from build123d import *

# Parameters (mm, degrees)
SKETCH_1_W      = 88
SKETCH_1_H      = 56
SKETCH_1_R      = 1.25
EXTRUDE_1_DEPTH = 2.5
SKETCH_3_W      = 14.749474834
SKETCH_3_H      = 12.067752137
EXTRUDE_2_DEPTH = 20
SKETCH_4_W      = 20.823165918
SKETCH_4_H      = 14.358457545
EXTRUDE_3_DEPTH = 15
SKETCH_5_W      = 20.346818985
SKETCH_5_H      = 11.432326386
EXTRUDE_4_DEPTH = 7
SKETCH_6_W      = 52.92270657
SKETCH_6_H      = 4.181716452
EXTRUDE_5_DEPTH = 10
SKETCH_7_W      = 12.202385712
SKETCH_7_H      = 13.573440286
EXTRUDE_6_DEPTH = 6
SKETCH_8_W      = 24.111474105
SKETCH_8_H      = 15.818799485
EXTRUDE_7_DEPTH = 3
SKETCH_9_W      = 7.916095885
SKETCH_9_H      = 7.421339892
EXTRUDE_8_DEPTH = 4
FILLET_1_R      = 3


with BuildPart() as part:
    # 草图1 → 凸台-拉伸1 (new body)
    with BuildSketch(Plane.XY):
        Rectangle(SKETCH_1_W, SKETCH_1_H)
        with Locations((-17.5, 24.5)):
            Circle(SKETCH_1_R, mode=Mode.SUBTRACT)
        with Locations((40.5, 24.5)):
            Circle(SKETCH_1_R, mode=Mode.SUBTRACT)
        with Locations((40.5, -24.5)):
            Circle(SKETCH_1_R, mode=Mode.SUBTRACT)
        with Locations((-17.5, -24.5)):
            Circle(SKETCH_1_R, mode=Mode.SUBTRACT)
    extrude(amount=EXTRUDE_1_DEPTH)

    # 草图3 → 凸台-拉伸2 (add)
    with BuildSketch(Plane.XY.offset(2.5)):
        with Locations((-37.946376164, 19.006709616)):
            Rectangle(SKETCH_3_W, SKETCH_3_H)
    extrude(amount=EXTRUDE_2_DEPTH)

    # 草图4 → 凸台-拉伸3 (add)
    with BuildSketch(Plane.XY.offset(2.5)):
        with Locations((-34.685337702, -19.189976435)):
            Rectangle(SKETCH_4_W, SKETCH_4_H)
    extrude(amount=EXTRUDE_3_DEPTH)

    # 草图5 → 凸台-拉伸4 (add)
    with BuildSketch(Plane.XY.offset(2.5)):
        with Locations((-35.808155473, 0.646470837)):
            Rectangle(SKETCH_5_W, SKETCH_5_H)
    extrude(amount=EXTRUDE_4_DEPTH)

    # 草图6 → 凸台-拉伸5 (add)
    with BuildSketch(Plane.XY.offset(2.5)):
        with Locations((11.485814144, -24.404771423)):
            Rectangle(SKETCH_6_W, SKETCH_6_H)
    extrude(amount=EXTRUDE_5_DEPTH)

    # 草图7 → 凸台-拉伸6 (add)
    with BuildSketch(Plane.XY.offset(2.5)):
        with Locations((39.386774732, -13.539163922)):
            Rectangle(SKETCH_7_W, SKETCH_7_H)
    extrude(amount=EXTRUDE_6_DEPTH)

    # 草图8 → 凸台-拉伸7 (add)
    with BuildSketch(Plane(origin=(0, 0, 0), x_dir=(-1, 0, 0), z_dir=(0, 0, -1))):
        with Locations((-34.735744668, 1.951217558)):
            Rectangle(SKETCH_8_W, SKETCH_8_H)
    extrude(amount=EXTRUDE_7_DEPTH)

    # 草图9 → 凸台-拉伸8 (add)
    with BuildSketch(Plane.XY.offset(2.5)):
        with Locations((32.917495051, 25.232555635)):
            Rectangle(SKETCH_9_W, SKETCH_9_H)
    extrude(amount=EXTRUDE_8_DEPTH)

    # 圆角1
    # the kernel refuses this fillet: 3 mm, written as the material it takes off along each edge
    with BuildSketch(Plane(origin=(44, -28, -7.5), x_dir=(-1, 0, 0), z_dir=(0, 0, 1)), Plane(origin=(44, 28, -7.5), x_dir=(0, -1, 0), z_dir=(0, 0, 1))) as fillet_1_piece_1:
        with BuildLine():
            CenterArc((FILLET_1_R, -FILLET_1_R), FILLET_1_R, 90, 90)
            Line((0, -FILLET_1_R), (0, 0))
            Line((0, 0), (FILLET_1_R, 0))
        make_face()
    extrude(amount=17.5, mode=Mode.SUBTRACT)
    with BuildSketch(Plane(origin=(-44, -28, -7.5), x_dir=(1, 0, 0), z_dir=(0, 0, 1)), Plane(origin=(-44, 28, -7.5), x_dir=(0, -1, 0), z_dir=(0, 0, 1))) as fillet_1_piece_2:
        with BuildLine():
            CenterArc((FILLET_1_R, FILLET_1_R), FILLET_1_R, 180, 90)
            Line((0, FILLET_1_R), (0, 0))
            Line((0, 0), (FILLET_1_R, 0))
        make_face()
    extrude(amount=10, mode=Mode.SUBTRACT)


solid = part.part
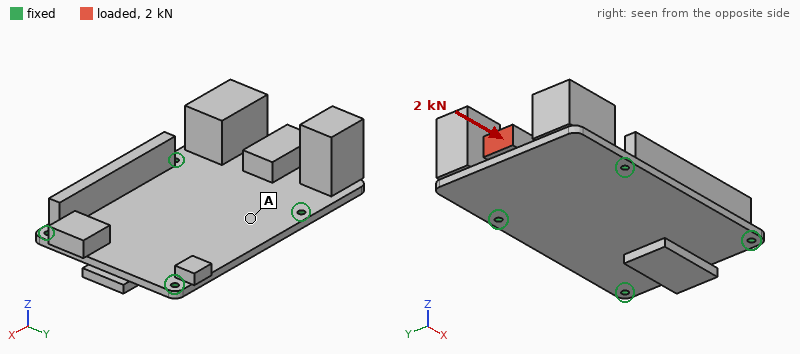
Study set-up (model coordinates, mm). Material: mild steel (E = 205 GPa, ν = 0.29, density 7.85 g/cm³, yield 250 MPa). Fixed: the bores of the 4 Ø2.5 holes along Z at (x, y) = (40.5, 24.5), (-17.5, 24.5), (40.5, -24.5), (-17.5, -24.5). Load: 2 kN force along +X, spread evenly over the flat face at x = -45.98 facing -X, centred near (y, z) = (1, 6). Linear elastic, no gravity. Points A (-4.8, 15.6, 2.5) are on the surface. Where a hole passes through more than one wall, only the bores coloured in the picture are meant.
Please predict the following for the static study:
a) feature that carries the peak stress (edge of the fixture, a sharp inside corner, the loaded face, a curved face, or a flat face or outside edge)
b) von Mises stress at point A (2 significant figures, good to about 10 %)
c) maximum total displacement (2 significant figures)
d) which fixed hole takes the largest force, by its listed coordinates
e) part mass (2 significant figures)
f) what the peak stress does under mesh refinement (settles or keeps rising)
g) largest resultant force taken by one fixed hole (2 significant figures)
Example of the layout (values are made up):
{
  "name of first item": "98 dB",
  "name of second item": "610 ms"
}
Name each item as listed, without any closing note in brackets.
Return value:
{
  "feature that carries the peak stress": "edge of the fixture",
  "von Mises stress at point A": "29 MPa",
  "maximum total displacement": "0.26 mm",
  "which fixed hole takes the largest force, by its listed coordinates": "(-17.5, 24.5)",
  "part mass": "210 g",
  "what the peak stress does under mesh refinement": "keeps rising",
  "largest resultant force taken by one fixed hole": "800 N"
}
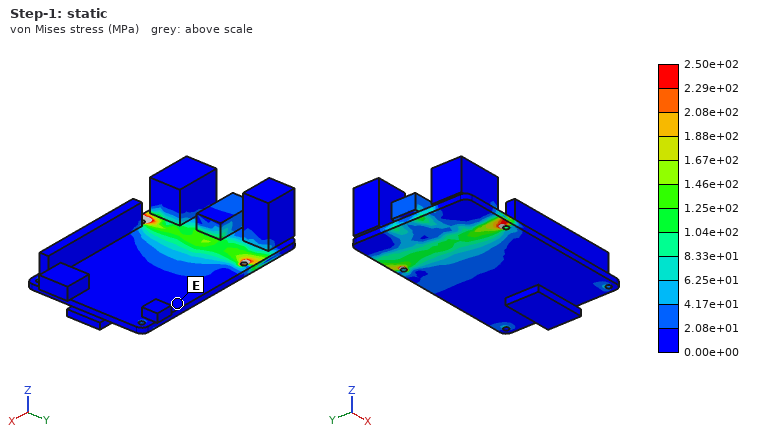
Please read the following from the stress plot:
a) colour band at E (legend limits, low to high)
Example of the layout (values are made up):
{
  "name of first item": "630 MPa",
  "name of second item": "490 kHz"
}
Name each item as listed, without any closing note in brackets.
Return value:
{
  "colour band at E": "0.00e+00 to 2.08e+01 MPa"
}
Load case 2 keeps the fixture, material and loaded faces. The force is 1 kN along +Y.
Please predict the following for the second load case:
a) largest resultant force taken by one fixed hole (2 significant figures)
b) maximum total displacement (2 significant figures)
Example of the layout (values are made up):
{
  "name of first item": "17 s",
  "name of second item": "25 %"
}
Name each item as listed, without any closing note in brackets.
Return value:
{
  "largest resultant force taken by one fixed hole": "750 N",
  "maximum total displacement": "22 µm"
}
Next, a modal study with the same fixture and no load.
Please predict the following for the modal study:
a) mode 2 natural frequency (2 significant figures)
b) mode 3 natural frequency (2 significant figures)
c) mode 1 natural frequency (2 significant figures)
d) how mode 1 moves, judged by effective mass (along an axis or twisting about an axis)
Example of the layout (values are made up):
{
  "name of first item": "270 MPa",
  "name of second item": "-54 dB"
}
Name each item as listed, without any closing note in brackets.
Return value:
{
  "mode 2 natural frequency": "2200 Hz",
  "mode 3 natural frequency": "2800 Hz",
  "mode 1 natural frequency": "930 Hz",
  "how mode 1 moves, judged by effective mass": "along Z"
}
